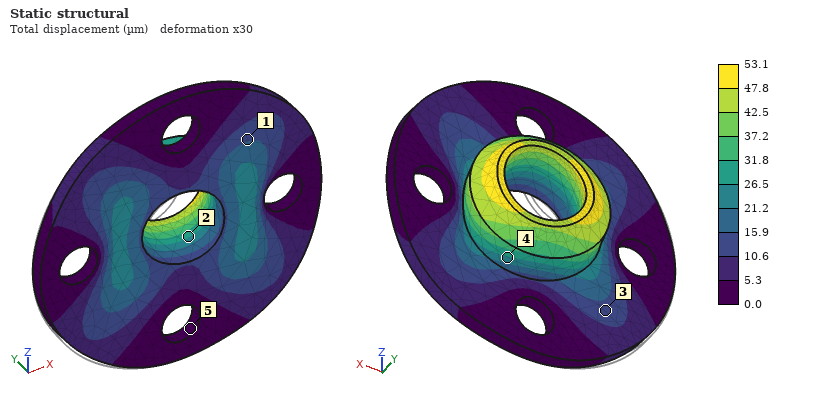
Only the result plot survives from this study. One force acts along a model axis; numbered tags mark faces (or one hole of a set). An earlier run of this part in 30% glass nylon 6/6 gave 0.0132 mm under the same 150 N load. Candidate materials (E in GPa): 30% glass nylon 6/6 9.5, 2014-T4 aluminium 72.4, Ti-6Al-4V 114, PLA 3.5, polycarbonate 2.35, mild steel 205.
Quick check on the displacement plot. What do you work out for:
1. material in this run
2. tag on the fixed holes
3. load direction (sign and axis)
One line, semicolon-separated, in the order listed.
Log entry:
polycarbonate; 5; +X
